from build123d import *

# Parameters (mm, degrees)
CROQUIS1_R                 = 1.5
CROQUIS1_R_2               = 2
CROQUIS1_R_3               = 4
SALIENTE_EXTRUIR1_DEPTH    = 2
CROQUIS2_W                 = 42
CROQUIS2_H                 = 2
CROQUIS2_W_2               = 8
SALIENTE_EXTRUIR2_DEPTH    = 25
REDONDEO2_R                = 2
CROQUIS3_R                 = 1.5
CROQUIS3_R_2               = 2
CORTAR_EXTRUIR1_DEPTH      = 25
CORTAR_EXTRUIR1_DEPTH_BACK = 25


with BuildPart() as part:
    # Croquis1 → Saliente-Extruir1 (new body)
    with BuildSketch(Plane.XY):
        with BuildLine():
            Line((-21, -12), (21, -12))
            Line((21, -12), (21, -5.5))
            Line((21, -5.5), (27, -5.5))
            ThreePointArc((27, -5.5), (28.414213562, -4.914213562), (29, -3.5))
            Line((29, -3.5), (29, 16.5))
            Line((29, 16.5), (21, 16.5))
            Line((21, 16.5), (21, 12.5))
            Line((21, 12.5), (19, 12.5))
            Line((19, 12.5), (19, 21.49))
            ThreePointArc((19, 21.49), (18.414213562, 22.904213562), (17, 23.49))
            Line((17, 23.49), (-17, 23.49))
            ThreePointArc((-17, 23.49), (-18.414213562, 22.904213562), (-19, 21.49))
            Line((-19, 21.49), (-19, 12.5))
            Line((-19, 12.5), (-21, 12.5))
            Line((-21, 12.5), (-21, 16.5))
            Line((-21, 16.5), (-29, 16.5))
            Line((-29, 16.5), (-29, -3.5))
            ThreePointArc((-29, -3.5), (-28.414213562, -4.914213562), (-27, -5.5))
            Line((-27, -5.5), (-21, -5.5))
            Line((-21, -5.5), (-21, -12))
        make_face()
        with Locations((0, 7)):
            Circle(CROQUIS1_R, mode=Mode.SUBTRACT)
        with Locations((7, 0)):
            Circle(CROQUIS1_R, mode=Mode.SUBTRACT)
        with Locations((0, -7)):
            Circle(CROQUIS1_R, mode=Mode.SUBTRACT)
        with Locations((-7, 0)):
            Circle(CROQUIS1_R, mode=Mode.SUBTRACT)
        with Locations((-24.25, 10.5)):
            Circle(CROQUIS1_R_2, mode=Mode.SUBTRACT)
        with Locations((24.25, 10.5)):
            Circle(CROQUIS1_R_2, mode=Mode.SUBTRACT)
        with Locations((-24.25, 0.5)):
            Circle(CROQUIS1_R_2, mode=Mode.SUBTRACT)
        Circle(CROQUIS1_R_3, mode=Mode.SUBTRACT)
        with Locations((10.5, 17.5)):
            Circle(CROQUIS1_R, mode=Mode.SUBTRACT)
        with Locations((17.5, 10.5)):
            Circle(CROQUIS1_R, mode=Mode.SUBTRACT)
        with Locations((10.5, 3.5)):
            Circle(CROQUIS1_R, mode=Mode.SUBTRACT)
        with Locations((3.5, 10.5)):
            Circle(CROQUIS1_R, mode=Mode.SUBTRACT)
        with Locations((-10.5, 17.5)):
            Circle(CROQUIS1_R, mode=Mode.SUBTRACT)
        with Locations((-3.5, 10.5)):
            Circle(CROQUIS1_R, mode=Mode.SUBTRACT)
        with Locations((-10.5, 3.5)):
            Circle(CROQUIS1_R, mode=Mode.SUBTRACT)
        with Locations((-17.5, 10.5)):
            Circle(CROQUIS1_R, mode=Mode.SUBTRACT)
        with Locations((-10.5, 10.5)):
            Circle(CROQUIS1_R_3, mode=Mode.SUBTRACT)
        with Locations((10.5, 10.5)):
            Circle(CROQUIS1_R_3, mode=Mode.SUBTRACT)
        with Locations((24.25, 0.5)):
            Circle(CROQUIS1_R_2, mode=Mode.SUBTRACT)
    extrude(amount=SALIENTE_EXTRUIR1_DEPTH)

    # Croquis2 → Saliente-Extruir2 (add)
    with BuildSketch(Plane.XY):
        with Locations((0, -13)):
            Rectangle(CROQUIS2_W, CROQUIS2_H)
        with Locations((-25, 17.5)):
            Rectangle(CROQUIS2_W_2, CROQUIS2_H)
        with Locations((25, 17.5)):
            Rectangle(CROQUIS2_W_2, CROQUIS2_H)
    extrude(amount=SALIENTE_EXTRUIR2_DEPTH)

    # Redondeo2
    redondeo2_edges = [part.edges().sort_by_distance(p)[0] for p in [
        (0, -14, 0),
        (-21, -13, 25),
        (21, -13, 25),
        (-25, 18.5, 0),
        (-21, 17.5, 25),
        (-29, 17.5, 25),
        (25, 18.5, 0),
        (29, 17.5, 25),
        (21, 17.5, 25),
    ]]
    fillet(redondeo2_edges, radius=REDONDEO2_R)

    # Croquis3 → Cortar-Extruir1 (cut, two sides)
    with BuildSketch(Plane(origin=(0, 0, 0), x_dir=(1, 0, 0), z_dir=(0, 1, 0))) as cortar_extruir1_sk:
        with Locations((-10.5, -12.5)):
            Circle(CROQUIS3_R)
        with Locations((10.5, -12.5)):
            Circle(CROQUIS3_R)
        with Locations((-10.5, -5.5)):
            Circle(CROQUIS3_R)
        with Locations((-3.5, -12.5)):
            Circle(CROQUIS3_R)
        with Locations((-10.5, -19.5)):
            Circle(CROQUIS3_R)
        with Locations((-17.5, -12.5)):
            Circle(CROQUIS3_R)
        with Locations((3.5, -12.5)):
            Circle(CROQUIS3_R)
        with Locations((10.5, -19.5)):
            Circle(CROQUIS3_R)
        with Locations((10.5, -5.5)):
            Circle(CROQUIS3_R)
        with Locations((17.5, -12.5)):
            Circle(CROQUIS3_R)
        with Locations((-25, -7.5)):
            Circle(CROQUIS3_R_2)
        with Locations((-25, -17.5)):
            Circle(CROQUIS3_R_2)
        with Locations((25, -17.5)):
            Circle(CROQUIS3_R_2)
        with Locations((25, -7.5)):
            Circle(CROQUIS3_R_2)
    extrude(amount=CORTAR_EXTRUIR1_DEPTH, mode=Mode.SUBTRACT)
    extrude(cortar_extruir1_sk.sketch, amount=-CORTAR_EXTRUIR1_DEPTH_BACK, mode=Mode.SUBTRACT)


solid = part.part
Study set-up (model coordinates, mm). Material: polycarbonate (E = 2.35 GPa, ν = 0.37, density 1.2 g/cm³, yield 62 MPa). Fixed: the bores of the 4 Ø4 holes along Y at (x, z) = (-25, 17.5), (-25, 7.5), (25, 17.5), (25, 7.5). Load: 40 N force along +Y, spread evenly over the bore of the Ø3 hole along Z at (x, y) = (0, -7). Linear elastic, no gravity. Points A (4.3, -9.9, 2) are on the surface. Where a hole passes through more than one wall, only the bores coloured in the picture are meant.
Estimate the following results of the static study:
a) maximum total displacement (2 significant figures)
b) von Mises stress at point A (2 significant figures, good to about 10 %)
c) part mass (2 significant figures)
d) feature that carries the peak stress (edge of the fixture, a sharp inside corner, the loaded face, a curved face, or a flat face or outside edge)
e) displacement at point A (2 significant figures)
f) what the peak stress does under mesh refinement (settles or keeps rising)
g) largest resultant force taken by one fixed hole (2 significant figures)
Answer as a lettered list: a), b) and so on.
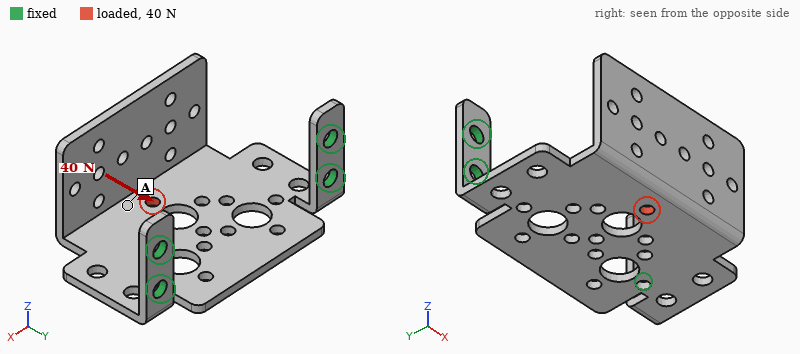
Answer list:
a) 0.72 mm
b) 1.5 MPa
c) 6.7 g
d) edge of the fixture
e) 0.54 mm
f) keeps rising
g) 21 N
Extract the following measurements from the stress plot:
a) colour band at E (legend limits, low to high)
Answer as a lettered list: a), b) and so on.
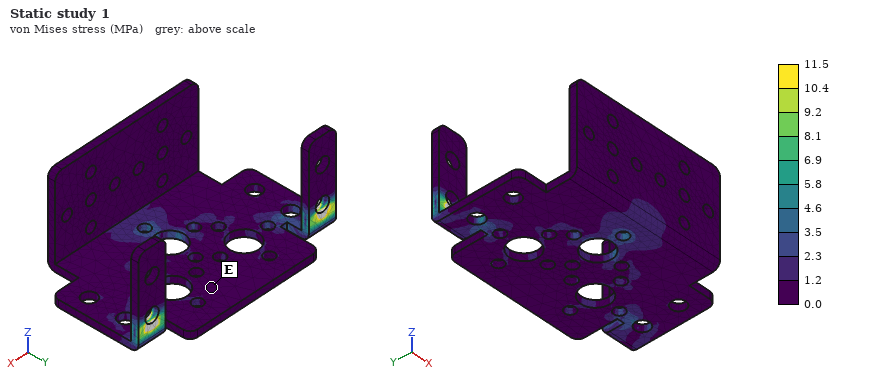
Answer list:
a) 0.0 to 1.2 MPa
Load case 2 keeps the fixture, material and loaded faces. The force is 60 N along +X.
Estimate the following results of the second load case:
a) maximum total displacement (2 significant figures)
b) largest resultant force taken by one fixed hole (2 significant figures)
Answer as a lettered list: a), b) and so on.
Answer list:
a) 0.50 mm
b) 43 N
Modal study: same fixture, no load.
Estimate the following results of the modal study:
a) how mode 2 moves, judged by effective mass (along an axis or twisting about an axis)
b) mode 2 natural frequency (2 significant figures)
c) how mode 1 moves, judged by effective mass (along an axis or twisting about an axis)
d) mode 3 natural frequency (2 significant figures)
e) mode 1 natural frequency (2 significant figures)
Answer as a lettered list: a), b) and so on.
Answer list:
a) along X
b) 350 Hz
c) along Z
d) 460 Hz
e) 110 Hz
